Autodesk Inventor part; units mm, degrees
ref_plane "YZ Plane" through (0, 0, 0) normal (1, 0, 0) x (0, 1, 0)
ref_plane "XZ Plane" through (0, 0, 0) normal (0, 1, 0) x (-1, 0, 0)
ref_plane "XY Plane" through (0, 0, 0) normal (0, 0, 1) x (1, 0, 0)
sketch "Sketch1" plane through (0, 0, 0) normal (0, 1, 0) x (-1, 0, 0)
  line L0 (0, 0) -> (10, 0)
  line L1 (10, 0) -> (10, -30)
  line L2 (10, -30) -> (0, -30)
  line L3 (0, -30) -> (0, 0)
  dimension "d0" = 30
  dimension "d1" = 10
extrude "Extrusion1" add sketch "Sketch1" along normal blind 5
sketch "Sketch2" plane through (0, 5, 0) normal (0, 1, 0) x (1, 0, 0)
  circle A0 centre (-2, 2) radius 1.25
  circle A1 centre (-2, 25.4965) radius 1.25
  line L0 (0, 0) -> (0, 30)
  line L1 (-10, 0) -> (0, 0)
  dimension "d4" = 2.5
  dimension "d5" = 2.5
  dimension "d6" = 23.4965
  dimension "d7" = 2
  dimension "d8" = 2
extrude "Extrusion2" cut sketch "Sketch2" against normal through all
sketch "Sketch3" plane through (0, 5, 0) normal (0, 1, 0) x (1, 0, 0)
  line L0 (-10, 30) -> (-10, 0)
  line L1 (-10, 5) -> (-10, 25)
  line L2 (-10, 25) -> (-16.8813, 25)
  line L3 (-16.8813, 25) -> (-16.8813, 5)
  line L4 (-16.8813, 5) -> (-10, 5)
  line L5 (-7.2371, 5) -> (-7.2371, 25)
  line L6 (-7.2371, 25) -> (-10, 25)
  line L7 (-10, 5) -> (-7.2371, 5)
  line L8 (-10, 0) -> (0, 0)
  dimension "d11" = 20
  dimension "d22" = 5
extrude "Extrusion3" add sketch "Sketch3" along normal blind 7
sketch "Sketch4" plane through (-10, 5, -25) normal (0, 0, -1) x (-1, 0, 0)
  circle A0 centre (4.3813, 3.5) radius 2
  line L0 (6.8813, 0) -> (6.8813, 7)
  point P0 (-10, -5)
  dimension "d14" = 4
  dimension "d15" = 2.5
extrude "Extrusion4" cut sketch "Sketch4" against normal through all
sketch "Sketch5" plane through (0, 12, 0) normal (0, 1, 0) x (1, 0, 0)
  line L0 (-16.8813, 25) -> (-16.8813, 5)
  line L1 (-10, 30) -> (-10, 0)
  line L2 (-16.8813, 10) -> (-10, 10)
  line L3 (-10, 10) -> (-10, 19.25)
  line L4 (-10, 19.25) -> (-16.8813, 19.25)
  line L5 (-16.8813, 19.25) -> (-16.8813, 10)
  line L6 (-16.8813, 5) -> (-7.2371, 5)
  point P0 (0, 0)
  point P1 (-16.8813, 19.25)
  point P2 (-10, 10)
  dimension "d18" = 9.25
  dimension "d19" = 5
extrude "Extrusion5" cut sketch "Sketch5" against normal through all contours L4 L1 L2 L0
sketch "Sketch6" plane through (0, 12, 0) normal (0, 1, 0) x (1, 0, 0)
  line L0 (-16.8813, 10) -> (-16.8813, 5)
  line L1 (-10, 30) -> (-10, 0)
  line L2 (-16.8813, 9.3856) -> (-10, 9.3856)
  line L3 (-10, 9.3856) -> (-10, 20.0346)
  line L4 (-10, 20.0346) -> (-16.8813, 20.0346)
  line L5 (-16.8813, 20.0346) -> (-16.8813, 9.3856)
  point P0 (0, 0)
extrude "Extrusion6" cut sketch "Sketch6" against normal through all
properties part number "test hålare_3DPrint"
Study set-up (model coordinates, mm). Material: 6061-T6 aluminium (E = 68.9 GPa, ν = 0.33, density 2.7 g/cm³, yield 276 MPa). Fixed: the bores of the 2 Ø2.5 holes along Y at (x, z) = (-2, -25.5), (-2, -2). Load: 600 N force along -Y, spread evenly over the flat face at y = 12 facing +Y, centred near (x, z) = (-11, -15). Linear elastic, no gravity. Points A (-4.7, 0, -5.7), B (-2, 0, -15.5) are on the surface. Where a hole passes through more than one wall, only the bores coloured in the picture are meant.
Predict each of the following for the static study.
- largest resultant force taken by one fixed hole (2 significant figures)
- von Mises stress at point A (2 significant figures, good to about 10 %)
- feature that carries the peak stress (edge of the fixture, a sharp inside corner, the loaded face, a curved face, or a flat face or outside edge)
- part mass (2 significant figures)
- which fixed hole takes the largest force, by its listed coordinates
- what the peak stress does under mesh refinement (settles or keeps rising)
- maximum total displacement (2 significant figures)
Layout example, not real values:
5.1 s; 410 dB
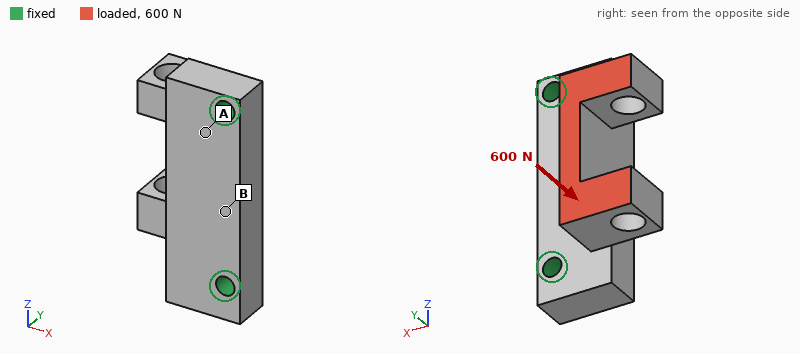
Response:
330 N; 38 MPa; edge of the fixture; 5.9 g; (-2, -25.5); keeps rising; 65 µm
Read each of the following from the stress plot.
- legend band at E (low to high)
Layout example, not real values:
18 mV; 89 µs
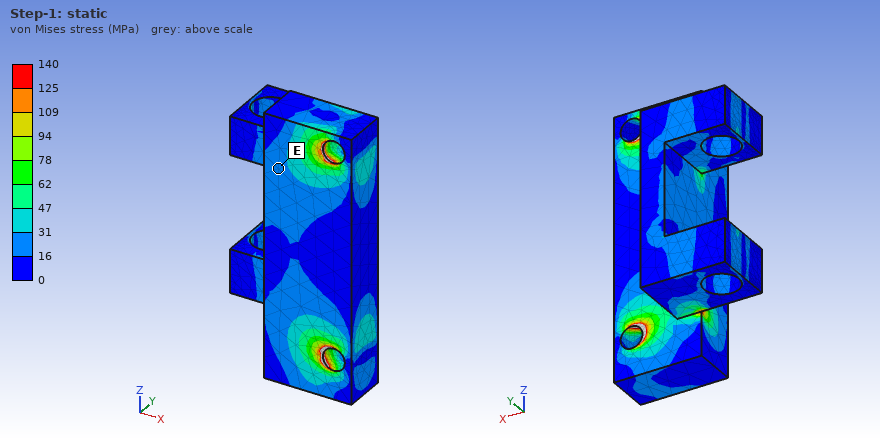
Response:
16 to 31 MPa
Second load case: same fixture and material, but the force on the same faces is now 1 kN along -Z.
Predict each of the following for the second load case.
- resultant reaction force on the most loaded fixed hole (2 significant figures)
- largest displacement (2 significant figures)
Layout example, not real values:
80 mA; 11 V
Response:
750 N; 43 µm
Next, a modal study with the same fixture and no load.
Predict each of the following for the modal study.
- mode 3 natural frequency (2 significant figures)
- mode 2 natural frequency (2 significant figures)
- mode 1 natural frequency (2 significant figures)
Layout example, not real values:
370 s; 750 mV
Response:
28 kHz; 18 kHz; 12 kHz
